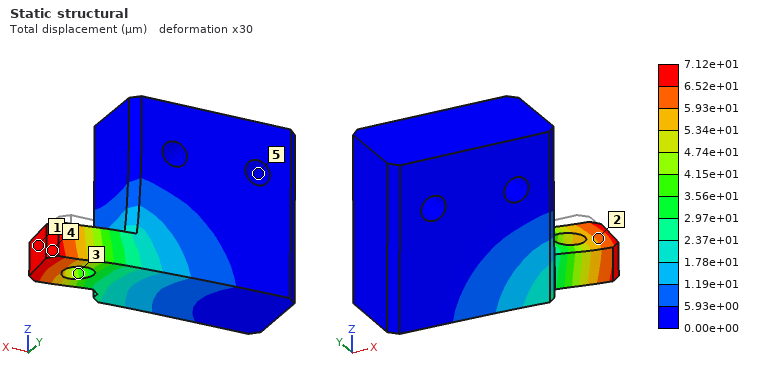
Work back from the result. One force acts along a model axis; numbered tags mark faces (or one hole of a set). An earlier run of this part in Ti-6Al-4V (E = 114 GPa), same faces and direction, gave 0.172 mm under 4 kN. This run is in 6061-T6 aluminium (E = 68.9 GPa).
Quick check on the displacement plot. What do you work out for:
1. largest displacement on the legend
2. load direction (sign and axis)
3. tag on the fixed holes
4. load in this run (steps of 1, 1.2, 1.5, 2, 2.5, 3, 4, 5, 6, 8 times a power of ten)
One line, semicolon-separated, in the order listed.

7.12e+01 µm; -Y; 5; 1 kN
